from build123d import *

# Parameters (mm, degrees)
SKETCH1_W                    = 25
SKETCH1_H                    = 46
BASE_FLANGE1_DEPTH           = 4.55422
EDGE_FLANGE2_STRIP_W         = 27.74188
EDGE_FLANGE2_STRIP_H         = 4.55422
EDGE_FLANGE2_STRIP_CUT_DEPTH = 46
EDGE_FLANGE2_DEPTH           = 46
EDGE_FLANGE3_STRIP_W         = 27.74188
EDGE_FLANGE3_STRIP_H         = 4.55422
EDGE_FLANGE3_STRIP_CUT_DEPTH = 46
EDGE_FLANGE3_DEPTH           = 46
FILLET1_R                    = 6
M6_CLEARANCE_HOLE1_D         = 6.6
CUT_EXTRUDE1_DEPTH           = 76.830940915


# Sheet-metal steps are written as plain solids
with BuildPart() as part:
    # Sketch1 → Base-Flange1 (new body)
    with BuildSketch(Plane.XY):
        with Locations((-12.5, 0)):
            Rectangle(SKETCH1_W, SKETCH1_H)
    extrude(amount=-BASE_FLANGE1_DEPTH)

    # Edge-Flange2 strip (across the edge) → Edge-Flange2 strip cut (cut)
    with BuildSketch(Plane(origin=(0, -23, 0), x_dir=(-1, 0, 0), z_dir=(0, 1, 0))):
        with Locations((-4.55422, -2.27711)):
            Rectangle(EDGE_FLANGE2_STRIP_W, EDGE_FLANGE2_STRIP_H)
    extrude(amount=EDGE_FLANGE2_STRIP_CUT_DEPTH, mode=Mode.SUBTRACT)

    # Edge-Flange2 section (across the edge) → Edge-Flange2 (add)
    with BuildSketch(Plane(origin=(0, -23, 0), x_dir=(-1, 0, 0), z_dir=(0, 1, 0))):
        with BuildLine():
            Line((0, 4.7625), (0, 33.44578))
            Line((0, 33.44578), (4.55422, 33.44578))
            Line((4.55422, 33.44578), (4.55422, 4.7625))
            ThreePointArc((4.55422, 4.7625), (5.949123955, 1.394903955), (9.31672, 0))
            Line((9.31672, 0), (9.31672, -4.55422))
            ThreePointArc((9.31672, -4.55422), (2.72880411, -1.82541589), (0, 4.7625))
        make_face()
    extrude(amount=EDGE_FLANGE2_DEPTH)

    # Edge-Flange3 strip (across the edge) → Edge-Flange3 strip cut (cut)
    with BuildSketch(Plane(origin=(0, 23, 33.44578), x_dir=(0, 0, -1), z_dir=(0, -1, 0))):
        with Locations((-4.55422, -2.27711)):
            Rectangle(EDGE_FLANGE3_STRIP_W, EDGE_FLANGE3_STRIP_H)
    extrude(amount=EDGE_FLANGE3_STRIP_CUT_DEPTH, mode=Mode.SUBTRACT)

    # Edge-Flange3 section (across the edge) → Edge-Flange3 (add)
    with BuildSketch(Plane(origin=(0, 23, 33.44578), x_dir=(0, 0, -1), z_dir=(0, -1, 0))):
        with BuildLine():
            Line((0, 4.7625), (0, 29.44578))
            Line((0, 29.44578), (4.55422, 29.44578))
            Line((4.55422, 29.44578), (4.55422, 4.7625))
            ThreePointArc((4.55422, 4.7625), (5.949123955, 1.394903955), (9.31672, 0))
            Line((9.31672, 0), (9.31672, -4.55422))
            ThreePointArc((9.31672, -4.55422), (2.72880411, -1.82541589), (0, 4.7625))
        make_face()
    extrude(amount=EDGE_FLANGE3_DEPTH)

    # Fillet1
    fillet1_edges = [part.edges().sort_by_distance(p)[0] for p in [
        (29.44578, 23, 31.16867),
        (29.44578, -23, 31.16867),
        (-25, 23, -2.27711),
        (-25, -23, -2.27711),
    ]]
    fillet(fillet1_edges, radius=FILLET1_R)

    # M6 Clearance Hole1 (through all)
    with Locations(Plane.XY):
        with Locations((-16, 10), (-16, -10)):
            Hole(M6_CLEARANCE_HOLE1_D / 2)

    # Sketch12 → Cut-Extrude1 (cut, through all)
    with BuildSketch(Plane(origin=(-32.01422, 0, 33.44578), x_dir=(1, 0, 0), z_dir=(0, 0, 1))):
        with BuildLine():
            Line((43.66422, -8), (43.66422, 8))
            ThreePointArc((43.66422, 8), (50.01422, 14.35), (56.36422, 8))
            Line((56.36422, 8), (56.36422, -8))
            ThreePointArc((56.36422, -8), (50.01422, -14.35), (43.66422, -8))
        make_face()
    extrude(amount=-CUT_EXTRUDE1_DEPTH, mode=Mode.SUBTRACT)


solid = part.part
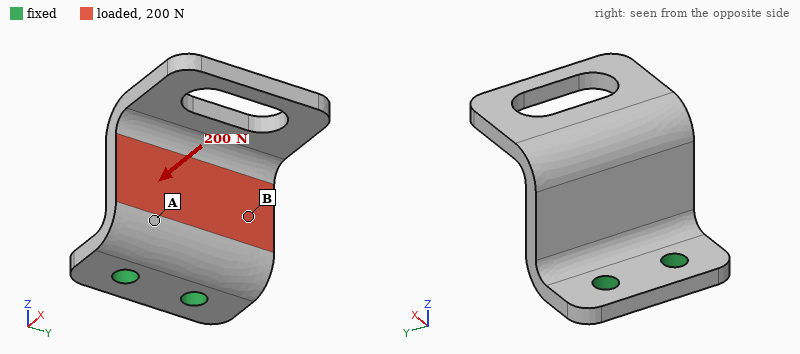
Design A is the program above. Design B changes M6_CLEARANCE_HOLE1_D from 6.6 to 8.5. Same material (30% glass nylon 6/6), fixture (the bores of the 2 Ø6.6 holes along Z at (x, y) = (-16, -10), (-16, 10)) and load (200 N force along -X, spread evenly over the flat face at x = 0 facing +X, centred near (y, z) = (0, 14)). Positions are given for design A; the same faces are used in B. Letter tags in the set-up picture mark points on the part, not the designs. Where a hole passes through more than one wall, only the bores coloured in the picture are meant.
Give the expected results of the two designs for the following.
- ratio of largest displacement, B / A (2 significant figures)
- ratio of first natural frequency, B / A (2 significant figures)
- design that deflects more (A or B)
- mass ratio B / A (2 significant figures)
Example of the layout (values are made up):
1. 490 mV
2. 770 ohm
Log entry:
1. 0.92
2. 1.0
3. A
4. 0.99
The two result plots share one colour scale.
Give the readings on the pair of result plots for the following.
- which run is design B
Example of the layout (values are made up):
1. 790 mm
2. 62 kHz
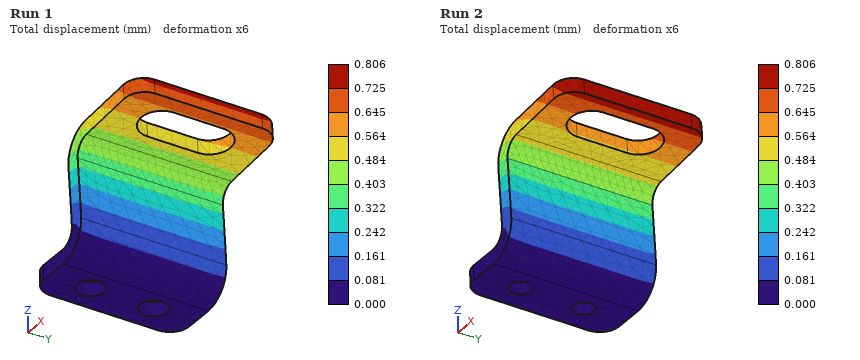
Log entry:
1. Run 1
